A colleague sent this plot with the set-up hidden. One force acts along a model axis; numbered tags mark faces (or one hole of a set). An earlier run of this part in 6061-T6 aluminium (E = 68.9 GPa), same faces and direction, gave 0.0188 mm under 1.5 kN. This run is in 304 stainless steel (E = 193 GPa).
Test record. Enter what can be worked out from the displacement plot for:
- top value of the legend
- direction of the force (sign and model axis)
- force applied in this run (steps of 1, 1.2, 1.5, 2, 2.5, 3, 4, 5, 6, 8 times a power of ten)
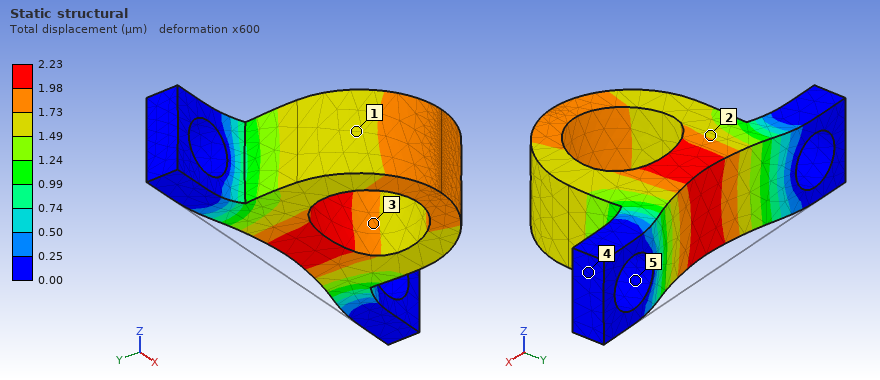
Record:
2.23 µm
-Y
500 N
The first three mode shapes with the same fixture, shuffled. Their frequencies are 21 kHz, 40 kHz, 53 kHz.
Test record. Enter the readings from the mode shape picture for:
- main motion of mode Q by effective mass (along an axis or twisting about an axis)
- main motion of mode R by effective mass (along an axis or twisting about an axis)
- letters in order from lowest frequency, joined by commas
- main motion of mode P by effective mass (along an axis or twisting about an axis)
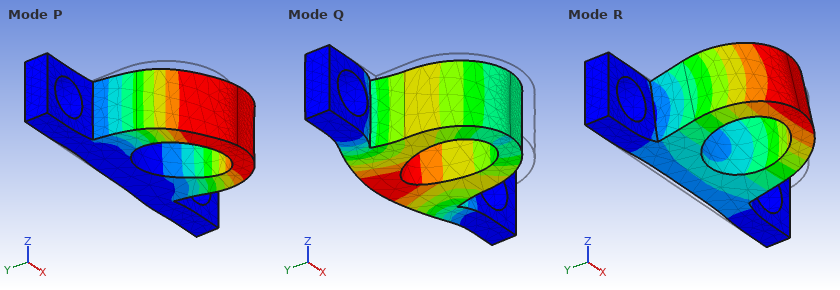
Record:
along Y
along Z
R, P, Q
along X
